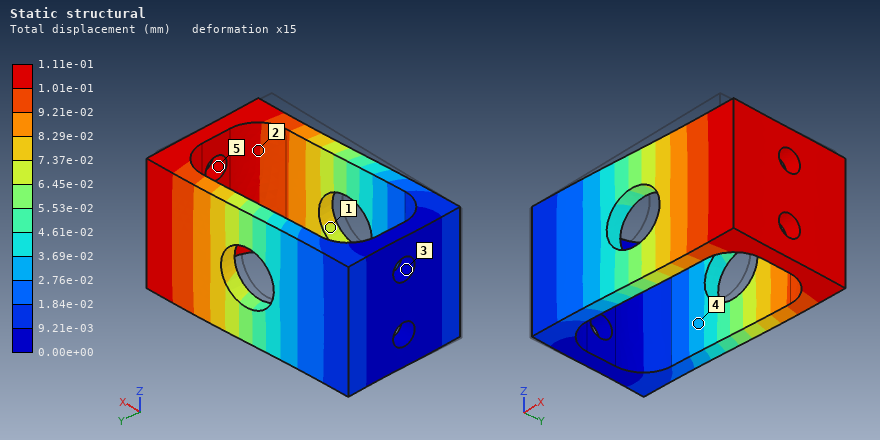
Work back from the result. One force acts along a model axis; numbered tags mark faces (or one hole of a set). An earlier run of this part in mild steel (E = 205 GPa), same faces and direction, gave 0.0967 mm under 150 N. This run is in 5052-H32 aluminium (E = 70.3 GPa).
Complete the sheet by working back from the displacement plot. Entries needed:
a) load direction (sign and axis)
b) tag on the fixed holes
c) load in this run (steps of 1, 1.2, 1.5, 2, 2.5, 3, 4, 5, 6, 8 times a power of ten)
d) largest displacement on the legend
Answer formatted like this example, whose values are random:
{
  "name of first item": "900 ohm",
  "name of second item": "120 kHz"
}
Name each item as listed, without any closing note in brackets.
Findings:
{
  "load direction": "+Y",
  "tag on the fixed holes": "3",
  "load in this run": "60 N",
  "largest displacement on the legend": "1.11e-01 mm"
}
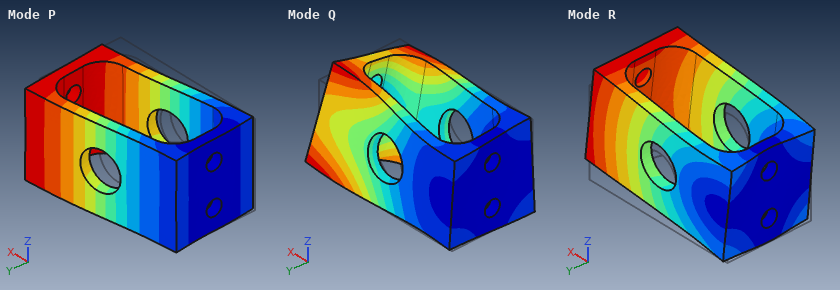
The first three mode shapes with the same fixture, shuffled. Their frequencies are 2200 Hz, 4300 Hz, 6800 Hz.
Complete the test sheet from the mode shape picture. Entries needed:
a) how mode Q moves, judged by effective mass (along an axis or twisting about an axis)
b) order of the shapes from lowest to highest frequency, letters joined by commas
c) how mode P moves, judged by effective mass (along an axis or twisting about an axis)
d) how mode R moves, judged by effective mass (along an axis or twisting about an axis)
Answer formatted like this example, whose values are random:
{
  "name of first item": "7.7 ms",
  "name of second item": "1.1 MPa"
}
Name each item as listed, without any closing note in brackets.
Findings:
{
  "how mode Q moves, judged by effective mass": "twisting about X",
  "order of the shapes from lowest to highest frequency, letters joined by commas": "P, R, Q",
  "how mode P moves, judged by effective mass": "along Y",
  "how mode R moves, judged by effective mass": "along Z"
}
